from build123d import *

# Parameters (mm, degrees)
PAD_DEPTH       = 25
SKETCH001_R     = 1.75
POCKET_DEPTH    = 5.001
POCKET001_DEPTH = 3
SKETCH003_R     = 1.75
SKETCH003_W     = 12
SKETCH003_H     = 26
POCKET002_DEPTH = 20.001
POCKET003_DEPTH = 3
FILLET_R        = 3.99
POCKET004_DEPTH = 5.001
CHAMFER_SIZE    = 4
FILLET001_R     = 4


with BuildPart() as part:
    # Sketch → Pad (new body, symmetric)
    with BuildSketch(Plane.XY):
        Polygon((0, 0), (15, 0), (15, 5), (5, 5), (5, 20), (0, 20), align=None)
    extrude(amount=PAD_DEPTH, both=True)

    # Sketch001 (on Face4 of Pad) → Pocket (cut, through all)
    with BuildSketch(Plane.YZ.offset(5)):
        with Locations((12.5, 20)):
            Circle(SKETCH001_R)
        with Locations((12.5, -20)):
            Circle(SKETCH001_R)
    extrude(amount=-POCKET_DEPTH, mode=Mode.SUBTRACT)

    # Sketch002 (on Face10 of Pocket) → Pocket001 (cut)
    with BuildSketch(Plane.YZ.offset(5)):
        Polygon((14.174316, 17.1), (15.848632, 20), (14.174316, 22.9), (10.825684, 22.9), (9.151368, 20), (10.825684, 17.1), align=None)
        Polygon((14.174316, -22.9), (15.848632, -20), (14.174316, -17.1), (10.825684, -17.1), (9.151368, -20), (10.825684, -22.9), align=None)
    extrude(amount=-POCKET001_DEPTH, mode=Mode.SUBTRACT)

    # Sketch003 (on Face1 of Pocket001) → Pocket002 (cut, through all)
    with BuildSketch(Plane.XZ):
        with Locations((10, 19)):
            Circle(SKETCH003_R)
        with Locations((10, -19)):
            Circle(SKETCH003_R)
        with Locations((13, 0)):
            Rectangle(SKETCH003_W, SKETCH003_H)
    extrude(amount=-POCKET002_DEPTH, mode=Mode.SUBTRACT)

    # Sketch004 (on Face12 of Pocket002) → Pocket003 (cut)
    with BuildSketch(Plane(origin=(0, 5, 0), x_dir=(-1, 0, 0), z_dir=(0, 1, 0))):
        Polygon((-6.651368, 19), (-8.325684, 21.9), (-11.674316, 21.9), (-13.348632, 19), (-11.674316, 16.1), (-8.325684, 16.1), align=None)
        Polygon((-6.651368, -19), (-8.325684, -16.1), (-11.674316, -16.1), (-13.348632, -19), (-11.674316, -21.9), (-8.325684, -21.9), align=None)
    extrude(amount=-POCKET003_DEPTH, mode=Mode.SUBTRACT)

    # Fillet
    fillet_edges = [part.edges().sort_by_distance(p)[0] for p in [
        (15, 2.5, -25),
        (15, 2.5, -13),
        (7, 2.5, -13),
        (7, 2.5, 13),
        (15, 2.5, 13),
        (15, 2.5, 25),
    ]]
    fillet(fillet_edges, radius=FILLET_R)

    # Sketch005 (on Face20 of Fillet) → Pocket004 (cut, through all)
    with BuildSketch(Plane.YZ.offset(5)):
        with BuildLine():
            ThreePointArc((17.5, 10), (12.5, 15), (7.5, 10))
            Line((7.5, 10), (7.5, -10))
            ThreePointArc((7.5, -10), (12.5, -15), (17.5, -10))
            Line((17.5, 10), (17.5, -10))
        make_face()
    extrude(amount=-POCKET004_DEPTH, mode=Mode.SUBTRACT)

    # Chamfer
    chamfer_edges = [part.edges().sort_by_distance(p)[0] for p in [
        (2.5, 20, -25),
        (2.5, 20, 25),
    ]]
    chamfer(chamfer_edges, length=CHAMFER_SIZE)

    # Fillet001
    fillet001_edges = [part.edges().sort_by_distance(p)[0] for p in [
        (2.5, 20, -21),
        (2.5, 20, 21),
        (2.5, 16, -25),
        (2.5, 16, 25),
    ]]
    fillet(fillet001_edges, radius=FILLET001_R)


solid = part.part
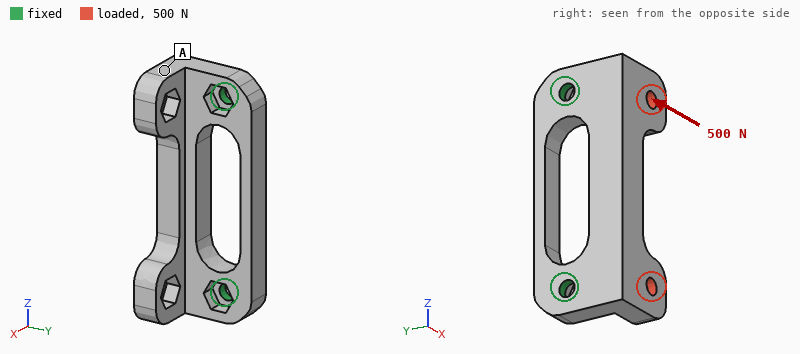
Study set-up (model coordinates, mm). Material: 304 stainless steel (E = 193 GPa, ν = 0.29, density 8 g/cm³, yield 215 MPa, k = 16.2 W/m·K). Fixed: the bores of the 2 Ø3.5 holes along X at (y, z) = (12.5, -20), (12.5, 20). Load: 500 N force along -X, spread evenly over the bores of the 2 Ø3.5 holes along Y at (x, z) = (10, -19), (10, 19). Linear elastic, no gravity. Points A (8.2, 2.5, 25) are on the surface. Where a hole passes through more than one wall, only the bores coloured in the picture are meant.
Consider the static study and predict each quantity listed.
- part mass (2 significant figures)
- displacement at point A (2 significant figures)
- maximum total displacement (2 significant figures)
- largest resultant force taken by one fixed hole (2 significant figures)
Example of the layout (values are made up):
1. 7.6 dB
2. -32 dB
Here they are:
1. 36 g
2. 19 µm
3. 32 µm
4. 250 N
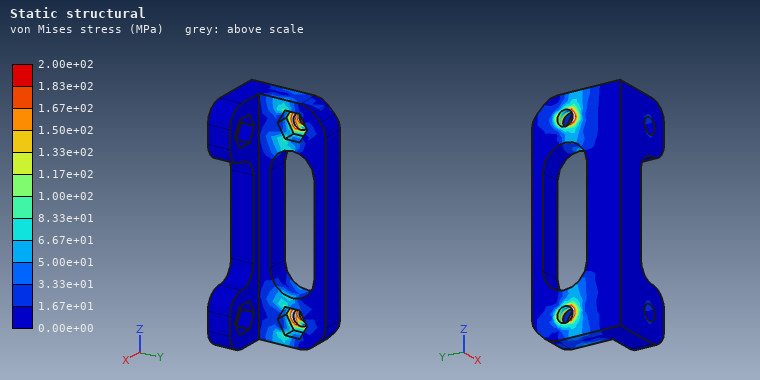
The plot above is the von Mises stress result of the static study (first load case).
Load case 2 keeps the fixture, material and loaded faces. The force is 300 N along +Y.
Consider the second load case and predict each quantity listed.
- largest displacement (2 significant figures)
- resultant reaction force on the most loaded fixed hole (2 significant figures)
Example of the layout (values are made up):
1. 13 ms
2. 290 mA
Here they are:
1. 19 µm
2. 150 N
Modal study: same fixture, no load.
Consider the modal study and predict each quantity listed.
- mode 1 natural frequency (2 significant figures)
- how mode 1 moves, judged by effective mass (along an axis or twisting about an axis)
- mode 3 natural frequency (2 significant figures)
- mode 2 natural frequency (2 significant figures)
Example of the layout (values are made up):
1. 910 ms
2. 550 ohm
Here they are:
1. 5300 Hz
2. along X
3. 11 kHz
4. 9200 Hz
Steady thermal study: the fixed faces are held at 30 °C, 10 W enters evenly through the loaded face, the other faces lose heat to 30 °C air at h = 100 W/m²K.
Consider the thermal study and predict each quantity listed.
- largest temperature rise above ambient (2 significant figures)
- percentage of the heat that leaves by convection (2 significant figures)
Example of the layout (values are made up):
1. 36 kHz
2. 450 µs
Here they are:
1. 70 K
2. 65 %
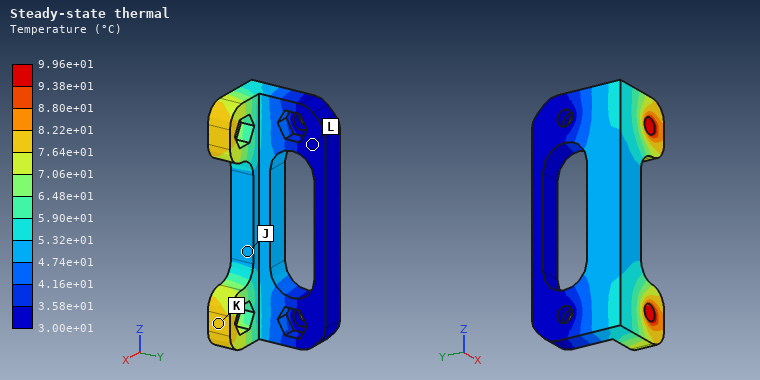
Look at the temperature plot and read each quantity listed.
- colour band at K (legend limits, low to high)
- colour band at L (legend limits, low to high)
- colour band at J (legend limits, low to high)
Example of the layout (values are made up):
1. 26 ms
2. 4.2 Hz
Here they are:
1. 7.64e+01 to 8.22e+01 °C
2. 3.00e+01 to 3.58e+01 °C
3. 4.74e+01 to 5.32e+01 °C
